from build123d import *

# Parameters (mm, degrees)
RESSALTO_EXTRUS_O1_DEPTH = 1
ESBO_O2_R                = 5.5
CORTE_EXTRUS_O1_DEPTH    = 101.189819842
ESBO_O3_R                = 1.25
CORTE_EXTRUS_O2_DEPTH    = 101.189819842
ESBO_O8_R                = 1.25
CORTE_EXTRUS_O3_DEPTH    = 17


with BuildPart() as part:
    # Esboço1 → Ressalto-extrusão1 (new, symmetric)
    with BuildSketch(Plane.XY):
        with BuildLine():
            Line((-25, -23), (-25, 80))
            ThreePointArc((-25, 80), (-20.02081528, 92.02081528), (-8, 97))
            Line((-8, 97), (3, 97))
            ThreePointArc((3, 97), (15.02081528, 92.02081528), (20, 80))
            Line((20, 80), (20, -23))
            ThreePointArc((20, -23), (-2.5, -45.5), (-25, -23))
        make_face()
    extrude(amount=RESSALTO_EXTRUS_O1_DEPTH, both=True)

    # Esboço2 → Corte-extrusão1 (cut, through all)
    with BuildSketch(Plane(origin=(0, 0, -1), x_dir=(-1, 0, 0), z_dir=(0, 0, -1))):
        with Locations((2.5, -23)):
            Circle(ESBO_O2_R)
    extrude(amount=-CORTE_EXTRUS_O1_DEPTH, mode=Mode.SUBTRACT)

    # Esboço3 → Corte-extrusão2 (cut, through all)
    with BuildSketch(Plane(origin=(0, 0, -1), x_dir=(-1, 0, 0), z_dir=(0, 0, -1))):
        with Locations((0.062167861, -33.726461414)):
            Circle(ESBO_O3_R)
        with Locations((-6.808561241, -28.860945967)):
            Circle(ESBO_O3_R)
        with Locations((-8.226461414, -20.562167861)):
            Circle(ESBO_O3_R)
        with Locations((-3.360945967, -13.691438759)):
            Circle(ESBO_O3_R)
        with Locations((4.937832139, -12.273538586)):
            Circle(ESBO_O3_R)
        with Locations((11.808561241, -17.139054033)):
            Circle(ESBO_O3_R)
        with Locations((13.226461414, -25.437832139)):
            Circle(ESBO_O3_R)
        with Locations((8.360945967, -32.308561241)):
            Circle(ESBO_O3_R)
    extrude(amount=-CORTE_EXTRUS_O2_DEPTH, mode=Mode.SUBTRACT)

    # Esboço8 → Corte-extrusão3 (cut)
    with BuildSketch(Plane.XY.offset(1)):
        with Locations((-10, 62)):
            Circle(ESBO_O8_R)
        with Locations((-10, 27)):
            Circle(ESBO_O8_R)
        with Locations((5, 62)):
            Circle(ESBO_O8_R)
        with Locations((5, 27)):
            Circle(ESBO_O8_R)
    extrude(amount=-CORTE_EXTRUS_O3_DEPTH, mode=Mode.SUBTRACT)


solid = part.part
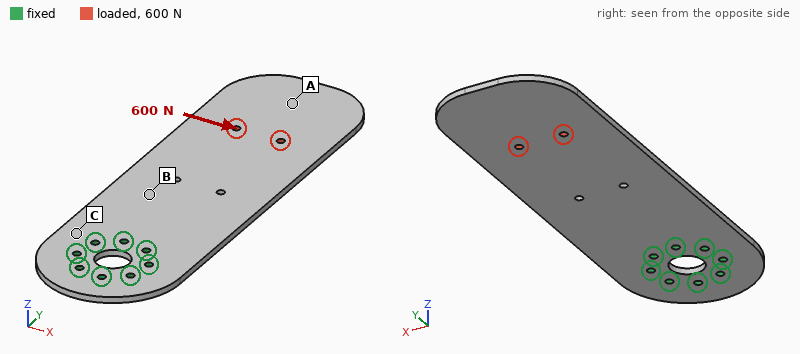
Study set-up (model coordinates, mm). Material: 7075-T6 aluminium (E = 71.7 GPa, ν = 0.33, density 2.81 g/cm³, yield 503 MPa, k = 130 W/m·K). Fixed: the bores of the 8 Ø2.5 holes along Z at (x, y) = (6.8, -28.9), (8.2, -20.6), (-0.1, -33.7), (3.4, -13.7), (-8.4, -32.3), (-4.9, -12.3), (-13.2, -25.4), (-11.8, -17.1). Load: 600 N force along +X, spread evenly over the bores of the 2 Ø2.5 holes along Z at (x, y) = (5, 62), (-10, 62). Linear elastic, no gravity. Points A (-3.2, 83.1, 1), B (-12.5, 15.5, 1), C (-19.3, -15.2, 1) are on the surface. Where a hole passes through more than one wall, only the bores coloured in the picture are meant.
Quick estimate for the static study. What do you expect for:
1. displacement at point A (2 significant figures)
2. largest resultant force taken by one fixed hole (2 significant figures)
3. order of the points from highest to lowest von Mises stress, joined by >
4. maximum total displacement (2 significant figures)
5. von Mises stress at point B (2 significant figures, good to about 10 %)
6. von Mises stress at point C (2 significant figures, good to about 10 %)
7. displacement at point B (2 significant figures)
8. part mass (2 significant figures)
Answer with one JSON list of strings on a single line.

["0.19 mm", "870 N", "C > B > A", "0.22 mm", "23 MPa", "42 MPa", "0.044 mm", "33 g"]
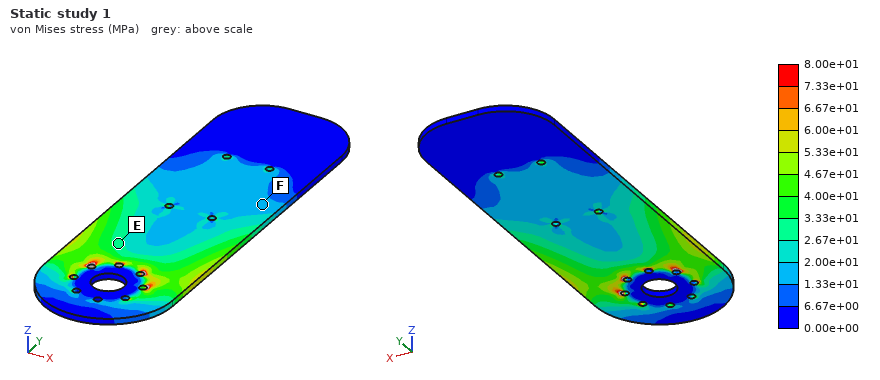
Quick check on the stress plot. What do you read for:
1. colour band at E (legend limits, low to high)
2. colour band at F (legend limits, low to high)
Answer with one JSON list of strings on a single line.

["2.67e+01 to 3.33e+01 MPa", "1.33e+01 to 2.00e+01 MPa"]
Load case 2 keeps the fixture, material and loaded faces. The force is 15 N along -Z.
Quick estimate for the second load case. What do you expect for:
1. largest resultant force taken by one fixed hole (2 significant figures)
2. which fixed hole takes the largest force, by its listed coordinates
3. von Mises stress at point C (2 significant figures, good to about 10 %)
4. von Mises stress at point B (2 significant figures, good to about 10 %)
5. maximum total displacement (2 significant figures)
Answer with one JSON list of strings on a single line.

["52 N", "(-4.9, -12.3)", "14 MPa", "22 MPa", "1.6 mm"]
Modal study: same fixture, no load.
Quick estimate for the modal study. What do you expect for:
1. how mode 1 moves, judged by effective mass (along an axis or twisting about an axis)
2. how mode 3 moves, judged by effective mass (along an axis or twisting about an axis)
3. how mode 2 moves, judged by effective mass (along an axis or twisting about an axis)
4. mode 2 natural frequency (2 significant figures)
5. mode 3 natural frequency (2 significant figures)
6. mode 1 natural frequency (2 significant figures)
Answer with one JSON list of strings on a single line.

["along Z", "along Z", "twisting about Y", "690 Hz", "870 Hz", "140 Hz"]
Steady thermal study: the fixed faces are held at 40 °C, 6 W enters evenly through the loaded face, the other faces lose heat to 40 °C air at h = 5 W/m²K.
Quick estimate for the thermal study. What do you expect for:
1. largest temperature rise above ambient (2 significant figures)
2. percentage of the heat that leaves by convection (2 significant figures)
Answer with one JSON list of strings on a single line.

["37 K", "19 %"]
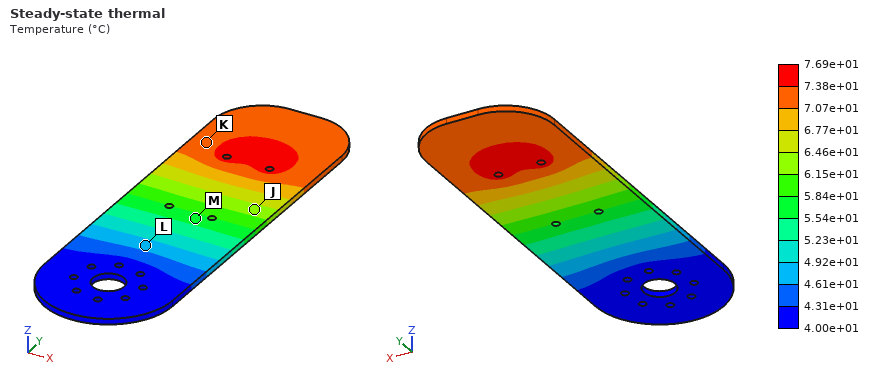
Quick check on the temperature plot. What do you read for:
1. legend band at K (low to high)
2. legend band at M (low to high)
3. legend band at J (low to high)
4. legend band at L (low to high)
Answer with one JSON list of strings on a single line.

["7.07e+01 to 7.38e+01 °C", "5.54e+01 to 5.84e+01 °C", "6.15e+01 to 6.46e+01 °C", "4.61e+01 to 4.92e+01 °C"]
